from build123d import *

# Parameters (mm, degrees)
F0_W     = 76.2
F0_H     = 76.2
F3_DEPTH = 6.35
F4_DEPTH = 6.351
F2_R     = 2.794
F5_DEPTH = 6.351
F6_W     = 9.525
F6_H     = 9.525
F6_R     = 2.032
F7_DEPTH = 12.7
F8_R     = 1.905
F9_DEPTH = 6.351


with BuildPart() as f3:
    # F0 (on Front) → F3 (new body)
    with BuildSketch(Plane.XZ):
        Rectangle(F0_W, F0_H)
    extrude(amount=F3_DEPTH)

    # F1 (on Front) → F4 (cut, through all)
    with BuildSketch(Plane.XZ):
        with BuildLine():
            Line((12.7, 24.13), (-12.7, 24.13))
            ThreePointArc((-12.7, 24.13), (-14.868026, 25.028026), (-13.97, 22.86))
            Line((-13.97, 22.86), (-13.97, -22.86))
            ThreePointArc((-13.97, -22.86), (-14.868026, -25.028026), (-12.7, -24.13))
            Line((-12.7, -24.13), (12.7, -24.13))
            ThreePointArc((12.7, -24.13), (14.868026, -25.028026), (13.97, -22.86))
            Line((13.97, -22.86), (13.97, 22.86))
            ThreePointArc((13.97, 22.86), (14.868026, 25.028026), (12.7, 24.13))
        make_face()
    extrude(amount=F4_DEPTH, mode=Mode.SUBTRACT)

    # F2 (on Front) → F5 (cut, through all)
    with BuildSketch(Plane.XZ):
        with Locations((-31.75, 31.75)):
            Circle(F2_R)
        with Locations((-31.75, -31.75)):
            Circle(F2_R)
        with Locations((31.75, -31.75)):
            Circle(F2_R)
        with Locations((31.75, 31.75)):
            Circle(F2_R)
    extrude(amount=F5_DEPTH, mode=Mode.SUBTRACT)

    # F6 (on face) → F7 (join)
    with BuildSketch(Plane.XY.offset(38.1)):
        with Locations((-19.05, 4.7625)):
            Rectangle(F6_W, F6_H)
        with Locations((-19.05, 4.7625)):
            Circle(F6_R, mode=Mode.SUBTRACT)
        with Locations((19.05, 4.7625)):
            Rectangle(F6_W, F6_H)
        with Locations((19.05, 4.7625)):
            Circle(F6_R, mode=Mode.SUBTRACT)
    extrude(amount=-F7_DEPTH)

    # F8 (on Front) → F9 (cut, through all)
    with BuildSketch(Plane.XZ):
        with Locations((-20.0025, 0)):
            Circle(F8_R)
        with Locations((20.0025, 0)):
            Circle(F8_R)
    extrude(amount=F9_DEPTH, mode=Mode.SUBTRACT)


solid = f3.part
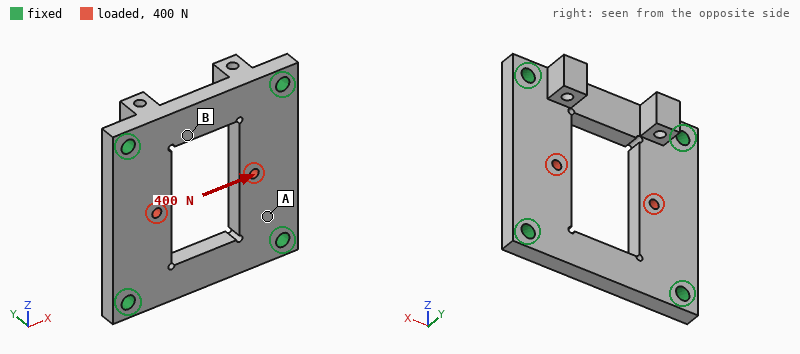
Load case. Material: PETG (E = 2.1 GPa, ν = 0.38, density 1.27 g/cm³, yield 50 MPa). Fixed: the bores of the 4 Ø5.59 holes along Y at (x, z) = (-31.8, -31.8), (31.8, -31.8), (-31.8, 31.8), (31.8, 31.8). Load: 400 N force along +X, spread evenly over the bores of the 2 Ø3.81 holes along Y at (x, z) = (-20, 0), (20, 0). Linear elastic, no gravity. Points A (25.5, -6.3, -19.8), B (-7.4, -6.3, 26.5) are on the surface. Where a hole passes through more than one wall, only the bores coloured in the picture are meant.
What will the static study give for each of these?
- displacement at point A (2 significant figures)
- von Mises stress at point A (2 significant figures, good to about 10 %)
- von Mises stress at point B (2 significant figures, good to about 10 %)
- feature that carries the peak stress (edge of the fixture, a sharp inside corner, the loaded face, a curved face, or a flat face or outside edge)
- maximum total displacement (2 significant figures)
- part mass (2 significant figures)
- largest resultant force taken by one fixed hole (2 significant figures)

21 µm
1.8 MPa
0.58 MPa
a curved face
61 µm
37 g
120 N
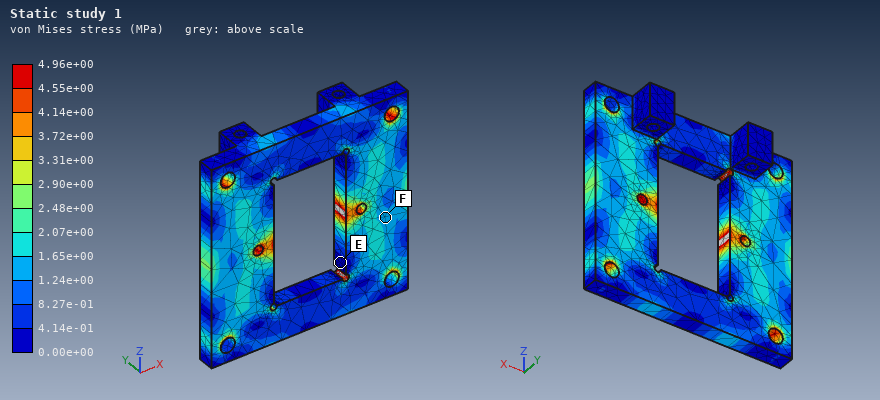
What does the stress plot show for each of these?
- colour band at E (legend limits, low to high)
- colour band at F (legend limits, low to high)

0.00e+00 to 4.14e-01 MPa
1.24e+00 to 1.65e+00 MPa
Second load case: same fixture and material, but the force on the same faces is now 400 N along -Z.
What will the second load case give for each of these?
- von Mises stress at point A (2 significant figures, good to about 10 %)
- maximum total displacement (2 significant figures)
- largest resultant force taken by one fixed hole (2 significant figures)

0.98 MPa
21 µm
100 N
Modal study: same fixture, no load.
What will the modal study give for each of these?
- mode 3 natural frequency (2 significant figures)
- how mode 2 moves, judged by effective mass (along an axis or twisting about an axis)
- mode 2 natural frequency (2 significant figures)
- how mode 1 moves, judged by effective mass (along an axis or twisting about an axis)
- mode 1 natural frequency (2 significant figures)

2100 Hz
twisting about Z
1900 Hz
along Y
1700 Hz
